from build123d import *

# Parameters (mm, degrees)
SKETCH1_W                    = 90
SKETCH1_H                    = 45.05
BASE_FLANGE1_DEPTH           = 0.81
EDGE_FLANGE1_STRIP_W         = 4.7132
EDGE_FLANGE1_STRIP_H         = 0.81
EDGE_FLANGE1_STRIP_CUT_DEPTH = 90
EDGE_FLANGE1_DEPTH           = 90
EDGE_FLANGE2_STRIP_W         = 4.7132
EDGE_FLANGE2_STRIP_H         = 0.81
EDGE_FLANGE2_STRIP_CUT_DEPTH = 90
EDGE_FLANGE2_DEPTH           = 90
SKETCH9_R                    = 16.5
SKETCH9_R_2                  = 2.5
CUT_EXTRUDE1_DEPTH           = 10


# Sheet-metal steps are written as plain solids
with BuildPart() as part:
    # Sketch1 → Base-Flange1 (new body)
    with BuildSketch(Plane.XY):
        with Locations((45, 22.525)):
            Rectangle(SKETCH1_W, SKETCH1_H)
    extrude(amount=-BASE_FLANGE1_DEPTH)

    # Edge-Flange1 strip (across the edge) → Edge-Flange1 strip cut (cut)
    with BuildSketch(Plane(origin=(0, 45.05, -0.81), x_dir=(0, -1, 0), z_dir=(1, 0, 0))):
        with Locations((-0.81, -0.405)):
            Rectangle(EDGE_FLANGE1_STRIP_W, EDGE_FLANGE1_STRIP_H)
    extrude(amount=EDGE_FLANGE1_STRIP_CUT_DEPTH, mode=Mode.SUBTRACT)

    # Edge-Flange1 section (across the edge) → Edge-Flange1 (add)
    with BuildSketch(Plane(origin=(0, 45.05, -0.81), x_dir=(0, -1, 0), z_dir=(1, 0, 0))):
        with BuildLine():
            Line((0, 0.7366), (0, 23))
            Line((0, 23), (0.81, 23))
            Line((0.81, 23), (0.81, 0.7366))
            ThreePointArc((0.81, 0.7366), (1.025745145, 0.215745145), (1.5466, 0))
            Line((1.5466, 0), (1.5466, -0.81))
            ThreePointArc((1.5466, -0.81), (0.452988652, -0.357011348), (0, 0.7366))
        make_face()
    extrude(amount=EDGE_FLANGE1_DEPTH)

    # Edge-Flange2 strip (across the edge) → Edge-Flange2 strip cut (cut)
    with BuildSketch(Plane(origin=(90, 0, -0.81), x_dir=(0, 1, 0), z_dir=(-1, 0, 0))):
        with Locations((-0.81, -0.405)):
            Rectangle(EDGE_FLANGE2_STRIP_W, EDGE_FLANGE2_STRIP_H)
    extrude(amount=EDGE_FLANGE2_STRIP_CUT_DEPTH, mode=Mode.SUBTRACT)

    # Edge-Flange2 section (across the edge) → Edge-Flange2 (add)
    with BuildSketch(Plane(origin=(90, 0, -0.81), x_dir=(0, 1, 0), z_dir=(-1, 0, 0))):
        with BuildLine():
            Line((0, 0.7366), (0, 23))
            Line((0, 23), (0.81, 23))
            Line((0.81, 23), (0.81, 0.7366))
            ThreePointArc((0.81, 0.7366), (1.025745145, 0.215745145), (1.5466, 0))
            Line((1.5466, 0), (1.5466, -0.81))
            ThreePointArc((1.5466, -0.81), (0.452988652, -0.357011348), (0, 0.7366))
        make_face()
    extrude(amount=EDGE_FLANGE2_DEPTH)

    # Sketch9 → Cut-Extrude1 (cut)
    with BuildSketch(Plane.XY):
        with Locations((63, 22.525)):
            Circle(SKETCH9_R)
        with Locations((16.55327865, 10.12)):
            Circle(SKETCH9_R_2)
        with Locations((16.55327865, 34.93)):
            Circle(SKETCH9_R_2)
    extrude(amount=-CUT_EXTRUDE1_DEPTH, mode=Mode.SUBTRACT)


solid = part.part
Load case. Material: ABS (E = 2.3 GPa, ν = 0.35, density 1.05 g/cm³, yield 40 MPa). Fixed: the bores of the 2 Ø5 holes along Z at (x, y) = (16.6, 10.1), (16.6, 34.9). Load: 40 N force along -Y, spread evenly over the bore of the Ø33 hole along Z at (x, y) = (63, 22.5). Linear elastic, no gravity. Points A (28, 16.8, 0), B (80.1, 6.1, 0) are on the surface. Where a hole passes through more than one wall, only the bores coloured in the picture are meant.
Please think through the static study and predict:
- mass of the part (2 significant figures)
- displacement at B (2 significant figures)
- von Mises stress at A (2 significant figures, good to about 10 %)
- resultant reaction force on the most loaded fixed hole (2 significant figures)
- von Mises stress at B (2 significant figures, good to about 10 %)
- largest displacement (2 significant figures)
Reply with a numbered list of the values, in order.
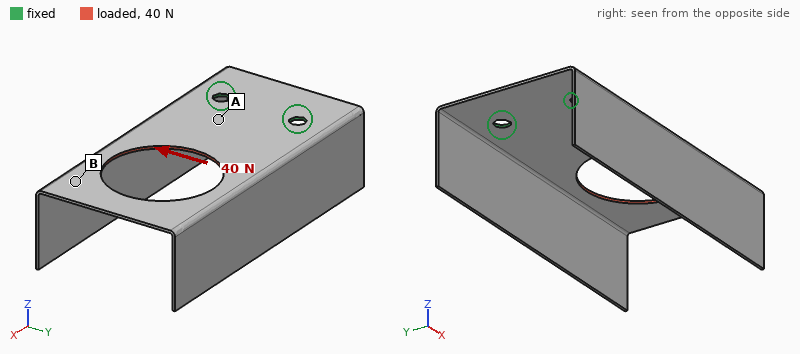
1. 6.1 g
2. 0.47 mm
3. 3.9 MPa
4. 69 N
5. 1.6 MPa
6. 0.58 mm
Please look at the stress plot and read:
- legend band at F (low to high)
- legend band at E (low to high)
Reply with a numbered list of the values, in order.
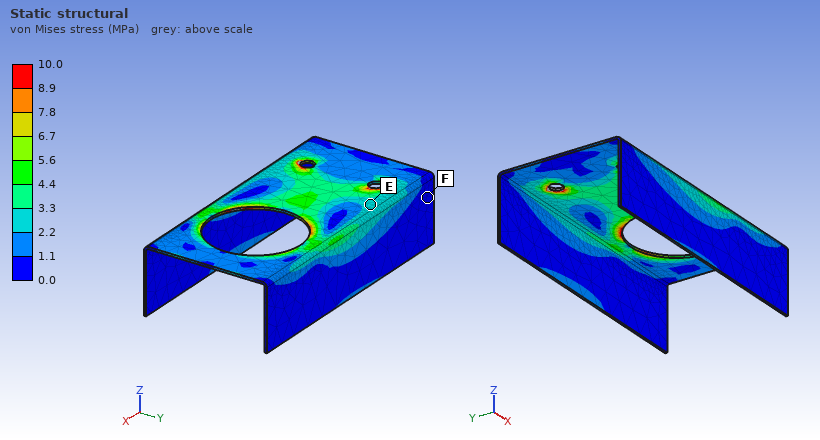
1. 0.0 to 1.1 MPa
2. 2.2 to 3.3 MPa
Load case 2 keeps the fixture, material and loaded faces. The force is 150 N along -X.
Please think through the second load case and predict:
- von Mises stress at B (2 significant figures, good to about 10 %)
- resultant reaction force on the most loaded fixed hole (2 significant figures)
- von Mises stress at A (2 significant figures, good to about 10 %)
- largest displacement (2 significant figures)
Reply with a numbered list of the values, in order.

1. 2.7 MPa
2. 75 N
3. 2.4 MPa
4. 0.41 mm
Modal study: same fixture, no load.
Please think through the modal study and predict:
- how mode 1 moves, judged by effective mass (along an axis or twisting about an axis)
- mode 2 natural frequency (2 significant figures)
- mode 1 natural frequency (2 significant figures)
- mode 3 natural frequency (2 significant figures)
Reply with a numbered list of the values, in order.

1. along Z
2. 84 Hz
3. 72 Hz
4. 150 Hz
